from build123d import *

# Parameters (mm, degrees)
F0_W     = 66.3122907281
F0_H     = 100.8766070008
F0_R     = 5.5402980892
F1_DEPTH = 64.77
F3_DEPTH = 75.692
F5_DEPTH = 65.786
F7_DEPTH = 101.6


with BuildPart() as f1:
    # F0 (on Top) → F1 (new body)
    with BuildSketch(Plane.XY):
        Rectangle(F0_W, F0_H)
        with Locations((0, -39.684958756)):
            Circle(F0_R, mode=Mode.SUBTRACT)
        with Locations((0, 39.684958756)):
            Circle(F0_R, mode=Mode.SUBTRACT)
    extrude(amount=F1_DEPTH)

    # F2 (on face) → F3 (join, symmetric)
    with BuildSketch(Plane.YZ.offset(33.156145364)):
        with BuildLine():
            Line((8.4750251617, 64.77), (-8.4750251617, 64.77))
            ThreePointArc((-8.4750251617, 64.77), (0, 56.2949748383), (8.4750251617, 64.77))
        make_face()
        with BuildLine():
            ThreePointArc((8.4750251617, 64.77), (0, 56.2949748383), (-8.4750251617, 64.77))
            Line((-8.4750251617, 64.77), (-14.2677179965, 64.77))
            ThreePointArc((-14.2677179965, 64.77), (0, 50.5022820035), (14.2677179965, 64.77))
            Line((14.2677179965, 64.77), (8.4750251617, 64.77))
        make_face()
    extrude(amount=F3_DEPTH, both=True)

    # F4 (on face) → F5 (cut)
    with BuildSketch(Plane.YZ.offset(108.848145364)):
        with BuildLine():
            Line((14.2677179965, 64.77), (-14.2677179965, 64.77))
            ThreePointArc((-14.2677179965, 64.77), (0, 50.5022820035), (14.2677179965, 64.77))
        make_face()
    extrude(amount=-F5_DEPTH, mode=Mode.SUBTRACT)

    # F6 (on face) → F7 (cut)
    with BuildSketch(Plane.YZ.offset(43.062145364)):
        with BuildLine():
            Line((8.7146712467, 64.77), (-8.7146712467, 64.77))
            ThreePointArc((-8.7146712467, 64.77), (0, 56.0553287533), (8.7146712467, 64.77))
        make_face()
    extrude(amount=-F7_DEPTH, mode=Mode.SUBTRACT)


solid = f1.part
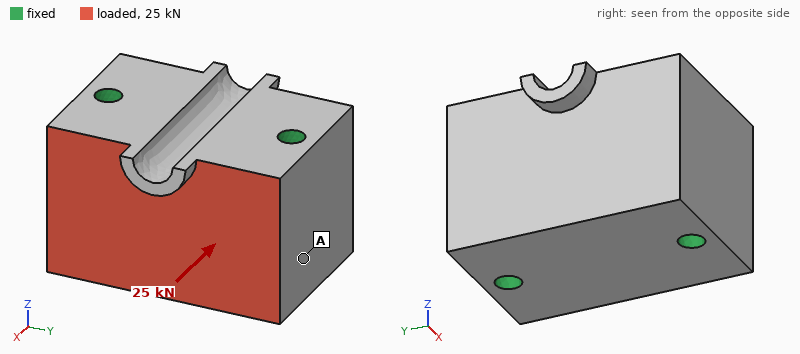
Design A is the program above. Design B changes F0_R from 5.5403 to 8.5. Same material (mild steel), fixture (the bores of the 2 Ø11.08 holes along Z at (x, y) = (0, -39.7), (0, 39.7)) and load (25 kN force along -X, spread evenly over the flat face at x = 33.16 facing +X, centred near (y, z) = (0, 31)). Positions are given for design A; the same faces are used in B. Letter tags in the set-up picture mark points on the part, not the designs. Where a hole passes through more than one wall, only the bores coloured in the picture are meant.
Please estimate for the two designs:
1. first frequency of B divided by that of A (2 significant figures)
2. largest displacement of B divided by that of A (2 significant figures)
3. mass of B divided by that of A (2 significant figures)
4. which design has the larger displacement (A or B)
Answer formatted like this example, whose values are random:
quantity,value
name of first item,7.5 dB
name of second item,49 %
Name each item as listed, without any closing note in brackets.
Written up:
quantity,value
first frequency of B divided by that of A,1.2
largest displacement of B divided by that of A,0.86
mass of B divided by that of A,0.96
which design has the larger displacement,A
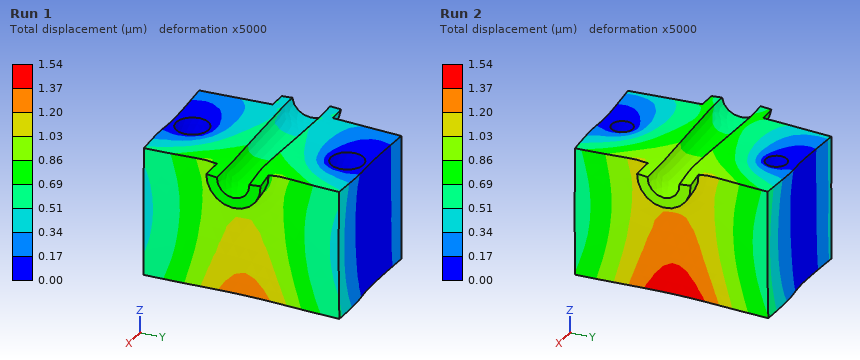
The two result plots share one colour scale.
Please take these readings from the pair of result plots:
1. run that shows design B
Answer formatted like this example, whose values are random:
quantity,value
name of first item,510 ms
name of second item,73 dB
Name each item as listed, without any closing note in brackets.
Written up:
quantity,value
run that shows design B,Run 1
